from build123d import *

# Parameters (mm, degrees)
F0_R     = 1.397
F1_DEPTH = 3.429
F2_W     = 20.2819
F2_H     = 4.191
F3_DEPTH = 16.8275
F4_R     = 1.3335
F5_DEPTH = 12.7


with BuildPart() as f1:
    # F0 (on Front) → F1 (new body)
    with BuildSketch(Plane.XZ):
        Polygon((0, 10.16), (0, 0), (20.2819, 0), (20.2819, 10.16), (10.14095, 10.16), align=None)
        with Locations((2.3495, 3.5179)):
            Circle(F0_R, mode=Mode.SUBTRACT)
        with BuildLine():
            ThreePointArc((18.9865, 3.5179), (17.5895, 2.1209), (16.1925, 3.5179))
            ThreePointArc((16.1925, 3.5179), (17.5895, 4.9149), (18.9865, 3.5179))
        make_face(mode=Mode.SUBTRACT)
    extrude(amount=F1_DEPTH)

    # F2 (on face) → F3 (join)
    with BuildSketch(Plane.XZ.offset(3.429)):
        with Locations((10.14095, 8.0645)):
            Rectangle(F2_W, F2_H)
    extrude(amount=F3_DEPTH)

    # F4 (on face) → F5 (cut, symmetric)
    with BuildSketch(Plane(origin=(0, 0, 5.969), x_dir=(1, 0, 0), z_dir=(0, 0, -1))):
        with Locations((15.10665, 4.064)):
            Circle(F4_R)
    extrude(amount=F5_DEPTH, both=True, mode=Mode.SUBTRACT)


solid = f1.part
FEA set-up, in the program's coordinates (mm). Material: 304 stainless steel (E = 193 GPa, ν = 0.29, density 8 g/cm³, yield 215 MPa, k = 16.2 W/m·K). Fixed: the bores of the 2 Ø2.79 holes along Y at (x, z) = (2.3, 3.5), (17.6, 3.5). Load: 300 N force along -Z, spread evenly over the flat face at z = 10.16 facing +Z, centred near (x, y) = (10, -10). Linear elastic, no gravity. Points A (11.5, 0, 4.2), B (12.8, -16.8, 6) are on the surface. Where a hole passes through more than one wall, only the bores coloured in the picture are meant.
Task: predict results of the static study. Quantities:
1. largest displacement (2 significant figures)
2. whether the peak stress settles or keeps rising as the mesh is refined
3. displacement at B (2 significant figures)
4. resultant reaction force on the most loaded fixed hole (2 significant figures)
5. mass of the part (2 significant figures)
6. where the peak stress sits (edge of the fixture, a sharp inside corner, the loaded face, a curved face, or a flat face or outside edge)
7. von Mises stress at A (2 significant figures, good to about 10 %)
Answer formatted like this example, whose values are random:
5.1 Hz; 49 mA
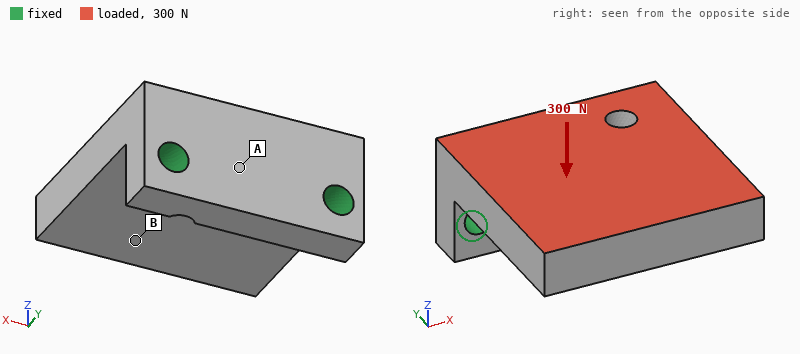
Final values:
24 µm; keeps rising; 19 µm; 160 N; 17 g; edge of the fixture; 25 MPa
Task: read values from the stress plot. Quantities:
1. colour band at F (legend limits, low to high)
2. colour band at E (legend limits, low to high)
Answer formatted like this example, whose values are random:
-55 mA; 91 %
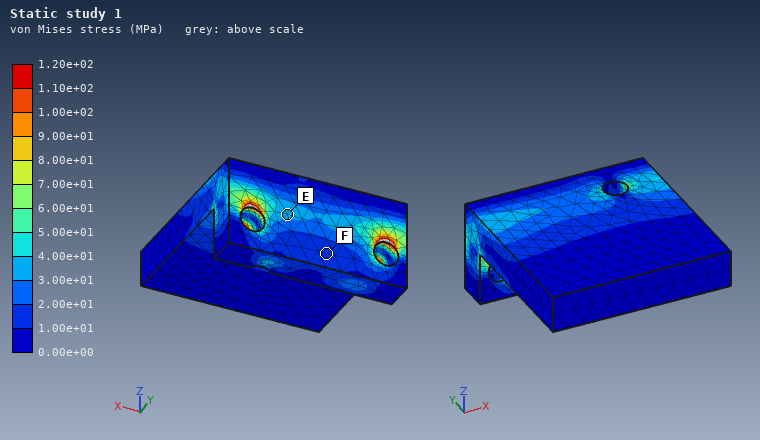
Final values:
1.00e+01 to 2.00e+01 MPa; 3.00e+01 to 4.00e+01 MPa
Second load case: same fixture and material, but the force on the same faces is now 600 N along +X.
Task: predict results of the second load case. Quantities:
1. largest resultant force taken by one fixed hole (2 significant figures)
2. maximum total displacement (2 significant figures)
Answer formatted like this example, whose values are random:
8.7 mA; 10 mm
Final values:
500 N; 5.2 µm
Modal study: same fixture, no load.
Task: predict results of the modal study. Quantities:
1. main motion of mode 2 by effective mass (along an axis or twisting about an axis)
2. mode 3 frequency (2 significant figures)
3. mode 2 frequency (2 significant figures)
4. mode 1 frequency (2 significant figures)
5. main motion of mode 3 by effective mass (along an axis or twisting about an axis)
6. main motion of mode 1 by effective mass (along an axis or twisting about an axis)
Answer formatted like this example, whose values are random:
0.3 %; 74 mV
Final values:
along X; 20 kHz; 15 kHz; 5900 Hz; along X; along Z
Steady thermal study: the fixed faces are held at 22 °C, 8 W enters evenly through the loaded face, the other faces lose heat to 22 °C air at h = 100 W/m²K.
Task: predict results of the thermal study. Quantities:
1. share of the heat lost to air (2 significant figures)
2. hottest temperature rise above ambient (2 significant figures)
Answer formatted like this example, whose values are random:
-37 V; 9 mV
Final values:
36 %; 51 K
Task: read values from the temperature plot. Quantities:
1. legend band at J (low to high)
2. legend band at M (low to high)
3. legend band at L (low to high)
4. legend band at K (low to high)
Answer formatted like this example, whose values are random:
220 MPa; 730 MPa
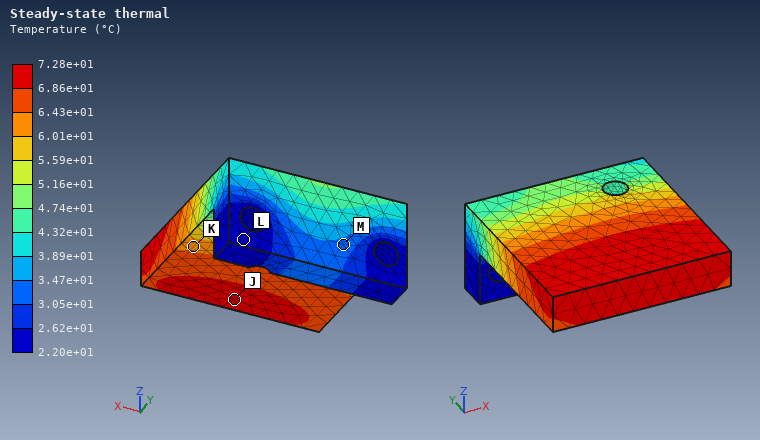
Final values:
6.86e+01 to 7.28e+01 °C; 3.05e+01 to 3.47e+01 °C; 2.20e+01 to 2.62e+01 °C; 6.01e+01 to 6.43e+01 °C
